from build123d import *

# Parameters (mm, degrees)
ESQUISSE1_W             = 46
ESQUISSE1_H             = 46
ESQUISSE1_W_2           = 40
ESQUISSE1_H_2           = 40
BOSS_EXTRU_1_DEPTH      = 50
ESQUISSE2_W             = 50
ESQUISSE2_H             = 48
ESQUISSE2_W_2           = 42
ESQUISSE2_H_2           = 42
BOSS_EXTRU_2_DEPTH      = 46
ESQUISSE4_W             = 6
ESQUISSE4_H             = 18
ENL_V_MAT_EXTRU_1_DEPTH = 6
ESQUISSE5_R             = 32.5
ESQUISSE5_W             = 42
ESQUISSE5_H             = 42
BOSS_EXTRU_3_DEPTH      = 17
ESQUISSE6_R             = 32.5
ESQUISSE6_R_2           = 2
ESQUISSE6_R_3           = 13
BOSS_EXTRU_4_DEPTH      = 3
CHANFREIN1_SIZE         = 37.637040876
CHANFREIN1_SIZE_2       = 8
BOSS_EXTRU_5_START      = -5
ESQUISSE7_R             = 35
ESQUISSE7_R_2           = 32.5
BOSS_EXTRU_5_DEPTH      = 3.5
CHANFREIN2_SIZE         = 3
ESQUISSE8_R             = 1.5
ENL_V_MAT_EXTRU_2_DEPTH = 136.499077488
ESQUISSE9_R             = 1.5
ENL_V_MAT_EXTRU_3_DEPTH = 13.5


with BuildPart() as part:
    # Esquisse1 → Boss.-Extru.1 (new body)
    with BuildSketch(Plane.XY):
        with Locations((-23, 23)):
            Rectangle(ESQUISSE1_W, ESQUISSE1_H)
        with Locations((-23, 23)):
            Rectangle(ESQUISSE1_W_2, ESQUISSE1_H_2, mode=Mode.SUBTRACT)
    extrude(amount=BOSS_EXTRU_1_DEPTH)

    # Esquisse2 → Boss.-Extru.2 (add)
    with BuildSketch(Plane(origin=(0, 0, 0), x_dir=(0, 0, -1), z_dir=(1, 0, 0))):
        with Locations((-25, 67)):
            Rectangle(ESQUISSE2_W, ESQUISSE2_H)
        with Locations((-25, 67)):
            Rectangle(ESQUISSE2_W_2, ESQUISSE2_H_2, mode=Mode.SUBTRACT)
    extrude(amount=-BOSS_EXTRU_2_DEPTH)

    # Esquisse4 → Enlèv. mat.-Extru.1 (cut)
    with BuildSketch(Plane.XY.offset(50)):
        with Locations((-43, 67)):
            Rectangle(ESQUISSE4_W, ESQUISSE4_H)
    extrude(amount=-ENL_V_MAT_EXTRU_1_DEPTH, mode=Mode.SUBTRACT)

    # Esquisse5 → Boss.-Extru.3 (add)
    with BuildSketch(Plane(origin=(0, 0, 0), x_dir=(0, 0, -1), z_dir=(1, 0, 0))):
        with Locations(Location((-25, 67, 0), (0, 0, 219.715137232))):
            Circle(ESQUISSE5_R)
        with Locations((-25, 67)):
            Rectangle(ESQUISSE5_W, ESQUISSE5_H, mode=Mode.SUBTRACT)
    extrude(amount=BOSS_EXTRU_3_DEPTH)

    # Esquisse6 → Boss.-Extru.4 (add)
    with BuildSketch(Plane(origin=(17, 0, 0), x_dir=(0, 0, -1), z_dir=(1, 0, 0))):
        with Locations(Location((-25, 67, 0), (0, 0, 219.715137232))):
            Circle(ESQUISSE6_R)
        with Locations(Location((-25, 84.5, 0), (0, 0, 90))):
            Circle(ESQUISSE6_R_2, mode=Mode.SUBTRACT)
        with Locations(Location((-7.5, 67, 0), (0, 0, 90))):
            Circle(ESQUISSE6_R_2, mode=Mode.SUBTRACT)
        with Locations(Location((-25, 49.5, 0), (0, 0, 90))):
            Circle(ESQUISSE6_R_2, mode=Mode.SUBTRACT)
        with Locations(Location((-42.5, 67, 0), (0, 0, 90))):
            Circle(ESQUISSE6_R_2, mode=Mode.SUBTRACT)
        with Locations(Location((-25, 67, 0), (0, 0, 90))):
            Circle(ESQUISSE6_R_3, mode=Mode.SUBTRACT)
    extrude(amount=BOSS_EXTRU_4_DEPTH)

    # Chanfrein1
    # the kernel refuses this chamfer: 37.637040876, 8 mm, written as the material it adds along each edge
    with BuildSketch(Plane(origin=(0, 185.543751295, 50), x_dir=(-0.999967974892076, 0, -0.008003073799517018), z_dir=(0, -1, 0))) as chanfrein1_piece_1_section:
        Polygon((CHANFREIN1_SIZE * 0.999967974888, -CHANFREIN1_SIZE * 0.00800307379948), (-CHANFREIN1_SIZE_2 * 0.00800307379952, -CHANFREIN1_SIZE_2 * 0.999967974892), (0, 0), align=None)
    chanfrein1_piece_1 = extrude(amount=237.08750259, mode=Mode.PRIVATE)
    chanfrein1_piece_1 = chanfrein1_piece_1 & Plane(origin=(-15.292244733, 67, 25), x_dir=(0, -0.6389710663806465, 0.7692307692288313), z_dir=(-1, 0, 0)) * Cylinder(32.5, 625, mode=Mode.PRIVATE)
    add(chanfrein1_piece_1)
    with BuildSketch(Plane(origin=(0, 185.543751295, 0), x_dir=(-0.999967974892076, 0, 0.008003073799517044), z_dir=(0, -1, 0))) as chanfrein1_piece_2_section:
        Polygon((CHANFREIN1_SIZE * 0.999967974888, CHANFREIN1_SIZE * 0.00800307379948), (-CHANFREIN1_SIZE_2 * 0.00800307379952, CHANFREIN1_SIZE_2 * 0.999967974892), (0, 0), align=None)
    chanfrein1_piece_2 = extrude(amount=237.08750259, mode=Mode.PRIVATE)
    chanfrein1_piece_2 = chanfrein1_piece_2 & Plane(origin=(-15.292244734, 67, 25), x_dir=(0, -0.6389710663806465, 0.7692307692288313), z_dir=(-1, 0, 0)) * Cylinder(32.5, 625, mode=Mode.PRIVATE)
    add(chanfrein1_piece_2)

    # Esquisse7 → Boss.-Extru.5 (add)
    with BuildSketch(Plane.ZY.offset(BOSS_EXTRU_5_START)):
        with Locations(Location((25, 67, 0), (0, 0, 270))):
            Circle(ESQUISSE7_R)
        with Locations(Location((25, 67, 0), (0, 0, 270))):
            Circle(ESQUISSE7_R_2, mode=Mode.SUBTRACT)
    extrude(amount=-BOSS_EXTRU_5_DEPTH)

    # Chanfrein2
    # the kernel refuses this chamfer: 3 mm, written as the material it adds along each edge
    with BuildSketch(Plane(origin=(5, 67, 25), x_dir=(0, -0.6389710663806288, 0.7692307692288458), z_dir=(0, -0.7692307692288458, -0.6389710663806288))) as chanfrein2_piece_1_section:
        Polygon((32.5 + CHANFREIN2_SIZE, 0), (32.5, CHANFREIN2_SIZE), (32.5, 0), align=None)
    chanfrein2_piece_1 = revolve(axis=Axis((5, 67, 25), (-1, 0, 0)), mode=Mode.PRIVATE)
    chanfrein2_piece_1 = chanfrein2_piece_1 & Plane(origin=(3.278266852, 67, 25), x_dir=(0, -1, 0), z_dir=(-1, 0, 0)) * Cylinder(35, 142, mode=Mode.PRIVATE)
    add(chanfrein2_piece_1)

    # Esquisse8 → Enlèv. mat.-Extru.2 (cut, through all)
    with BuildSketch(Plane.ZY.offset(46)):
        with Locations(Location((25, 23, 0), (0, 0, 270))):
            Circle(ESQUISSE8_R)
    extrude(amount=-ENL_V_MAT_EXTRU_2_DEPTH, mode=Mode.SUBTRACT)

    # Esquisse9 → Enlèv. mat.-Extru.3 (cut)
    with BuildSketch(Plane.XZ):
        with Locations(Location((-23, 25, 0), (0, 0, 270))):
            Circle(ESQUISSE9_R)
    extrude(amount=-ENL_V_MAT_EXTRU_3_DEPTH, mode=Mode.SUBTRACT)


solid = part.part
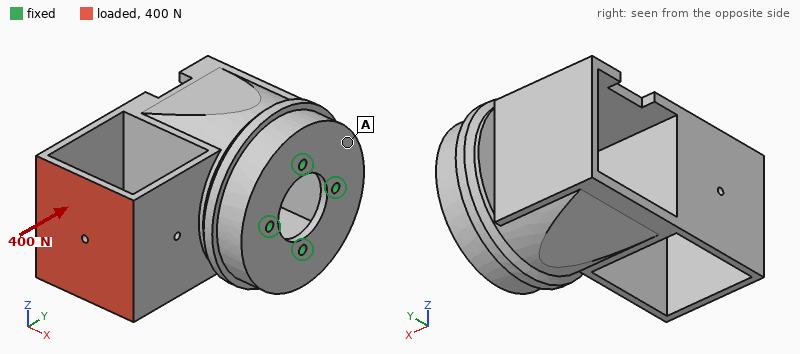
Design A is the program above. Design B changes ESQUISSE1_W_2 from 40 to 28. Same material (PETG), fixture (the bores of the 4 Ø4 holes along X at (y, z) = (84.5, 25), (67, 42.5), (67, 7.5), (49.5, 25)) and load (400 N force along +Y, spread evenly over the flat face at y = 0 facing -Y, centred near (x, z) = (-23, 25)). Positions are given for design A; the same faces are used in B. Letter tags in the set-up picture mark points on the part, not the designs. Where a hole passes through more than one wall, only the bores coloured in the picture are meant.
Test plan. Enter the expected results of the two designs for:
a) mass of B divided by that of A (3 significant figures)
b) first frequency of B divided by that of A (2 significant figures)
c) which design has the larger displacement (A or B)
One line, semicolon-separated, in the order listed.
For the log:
1.25; 1.1; A
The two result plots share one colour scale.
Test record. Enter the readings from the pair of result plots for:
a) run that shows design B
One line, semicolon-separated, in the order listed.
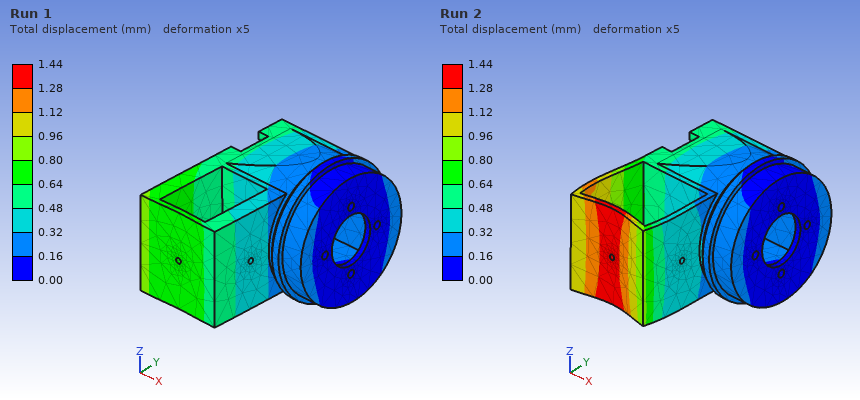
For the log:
Run 1
